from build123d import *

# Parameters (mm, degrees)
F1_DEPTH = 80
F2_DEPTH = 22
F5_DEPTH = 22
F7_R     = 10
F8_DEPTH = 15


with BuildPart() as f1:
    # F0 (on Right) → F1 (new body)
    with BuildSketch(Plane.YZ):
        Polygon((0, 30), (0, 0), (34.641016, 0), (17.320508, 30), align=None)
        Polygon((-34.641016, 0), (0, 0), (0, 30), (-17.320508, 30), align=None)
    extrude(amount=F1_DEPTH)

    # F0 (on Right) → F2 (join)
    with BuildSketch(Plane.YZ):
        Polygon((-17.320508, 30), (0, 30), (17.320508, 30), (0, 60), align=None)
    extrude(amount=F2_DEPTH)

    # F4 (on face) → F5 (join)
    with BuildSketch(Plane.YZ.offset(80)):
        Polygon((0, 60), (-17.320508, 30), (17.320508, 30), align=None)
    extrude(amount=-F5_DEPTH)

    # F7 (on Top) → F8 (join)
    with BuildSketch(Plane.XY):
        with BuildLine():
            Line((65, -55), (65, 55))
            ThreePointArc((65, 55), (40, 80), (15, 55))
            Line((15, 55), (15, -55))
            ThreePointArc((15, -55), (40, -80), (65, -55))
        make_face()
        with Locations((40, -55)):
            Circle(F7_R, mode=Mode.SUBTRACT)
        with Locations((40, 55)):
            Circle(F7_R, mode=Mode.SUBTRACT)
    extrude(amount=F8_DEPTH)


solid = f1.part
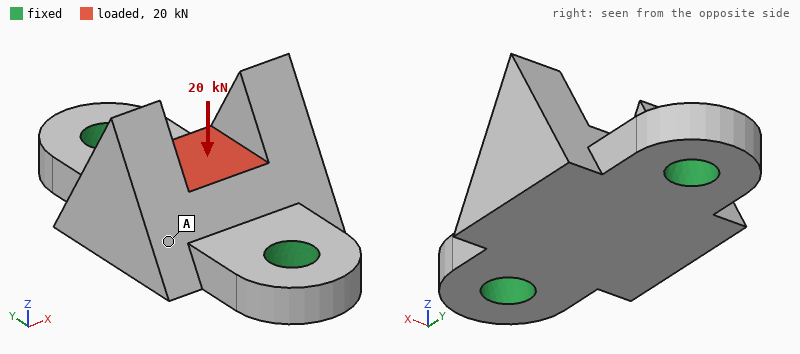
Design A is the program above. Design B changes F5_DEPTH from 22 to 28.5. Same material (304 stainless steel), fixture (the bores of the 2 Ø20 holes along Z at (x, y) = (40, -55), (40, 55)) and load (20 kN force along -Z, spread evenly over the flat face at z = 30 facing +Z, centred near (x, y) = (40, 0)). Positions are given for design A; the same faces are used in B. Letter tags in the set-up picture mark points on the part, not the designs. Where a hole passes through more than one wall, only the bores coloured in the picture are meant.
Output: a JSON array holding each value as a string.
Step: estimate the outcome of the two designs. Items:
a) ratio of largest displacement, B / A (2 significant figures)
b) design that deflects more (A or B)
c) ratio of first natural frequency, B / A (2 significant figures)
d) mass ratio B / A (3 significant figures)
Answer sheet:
["1.4", "B", "0.98", "1.02"]
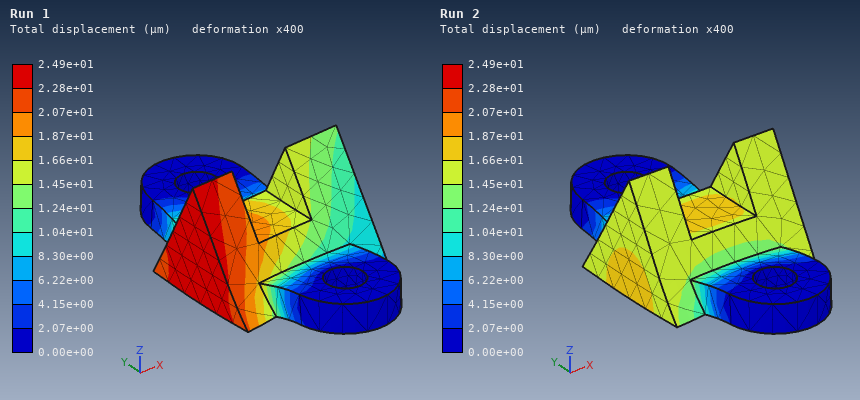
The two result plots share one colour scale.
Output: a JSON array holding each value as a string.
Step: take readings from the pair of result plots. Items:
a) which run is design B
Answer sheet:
["Run 1"]
